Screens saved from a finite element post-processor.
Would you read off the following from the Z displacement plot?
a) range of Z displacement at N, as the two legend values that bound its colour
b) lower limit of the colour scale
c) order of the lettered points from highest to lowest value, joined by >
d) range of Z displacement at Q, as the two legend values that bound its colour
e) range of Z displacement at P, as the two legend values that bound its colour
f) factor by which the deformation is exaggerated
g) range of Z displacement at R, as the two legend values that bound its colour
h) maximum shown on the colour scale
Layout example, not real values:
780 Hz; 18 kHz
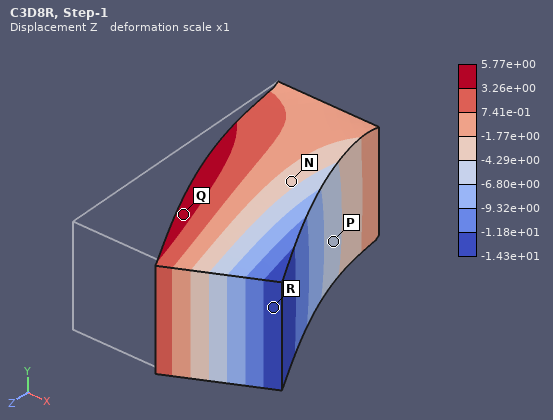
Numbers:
-4.29e+00 to -1.77e+00; -1.43e+01; Q > N > P > R; 3.26e+00 to 5.77e+00; -6.80e+00 to -4.29e+00; 1; -1.43e+01 to -1.18e+01; 5.77e+00
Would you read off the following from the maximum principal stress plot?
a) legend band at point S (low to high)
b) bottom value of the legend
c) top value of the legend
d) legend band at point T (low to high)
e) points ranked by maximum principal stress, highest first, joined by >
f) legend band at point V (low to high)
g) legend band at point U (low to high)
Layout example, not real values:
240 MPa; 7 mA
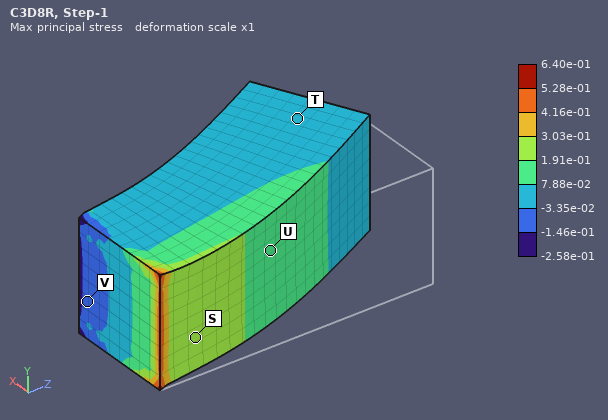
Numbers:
1.91e-01 to 3.03e-01; -2.58e-01; 6.40e-01; -3.35e-02 to 7.88e-02; S > U > T > V; -1.46e-01 to -3.35e-02; 7.88e-02 to 1.91e-01
